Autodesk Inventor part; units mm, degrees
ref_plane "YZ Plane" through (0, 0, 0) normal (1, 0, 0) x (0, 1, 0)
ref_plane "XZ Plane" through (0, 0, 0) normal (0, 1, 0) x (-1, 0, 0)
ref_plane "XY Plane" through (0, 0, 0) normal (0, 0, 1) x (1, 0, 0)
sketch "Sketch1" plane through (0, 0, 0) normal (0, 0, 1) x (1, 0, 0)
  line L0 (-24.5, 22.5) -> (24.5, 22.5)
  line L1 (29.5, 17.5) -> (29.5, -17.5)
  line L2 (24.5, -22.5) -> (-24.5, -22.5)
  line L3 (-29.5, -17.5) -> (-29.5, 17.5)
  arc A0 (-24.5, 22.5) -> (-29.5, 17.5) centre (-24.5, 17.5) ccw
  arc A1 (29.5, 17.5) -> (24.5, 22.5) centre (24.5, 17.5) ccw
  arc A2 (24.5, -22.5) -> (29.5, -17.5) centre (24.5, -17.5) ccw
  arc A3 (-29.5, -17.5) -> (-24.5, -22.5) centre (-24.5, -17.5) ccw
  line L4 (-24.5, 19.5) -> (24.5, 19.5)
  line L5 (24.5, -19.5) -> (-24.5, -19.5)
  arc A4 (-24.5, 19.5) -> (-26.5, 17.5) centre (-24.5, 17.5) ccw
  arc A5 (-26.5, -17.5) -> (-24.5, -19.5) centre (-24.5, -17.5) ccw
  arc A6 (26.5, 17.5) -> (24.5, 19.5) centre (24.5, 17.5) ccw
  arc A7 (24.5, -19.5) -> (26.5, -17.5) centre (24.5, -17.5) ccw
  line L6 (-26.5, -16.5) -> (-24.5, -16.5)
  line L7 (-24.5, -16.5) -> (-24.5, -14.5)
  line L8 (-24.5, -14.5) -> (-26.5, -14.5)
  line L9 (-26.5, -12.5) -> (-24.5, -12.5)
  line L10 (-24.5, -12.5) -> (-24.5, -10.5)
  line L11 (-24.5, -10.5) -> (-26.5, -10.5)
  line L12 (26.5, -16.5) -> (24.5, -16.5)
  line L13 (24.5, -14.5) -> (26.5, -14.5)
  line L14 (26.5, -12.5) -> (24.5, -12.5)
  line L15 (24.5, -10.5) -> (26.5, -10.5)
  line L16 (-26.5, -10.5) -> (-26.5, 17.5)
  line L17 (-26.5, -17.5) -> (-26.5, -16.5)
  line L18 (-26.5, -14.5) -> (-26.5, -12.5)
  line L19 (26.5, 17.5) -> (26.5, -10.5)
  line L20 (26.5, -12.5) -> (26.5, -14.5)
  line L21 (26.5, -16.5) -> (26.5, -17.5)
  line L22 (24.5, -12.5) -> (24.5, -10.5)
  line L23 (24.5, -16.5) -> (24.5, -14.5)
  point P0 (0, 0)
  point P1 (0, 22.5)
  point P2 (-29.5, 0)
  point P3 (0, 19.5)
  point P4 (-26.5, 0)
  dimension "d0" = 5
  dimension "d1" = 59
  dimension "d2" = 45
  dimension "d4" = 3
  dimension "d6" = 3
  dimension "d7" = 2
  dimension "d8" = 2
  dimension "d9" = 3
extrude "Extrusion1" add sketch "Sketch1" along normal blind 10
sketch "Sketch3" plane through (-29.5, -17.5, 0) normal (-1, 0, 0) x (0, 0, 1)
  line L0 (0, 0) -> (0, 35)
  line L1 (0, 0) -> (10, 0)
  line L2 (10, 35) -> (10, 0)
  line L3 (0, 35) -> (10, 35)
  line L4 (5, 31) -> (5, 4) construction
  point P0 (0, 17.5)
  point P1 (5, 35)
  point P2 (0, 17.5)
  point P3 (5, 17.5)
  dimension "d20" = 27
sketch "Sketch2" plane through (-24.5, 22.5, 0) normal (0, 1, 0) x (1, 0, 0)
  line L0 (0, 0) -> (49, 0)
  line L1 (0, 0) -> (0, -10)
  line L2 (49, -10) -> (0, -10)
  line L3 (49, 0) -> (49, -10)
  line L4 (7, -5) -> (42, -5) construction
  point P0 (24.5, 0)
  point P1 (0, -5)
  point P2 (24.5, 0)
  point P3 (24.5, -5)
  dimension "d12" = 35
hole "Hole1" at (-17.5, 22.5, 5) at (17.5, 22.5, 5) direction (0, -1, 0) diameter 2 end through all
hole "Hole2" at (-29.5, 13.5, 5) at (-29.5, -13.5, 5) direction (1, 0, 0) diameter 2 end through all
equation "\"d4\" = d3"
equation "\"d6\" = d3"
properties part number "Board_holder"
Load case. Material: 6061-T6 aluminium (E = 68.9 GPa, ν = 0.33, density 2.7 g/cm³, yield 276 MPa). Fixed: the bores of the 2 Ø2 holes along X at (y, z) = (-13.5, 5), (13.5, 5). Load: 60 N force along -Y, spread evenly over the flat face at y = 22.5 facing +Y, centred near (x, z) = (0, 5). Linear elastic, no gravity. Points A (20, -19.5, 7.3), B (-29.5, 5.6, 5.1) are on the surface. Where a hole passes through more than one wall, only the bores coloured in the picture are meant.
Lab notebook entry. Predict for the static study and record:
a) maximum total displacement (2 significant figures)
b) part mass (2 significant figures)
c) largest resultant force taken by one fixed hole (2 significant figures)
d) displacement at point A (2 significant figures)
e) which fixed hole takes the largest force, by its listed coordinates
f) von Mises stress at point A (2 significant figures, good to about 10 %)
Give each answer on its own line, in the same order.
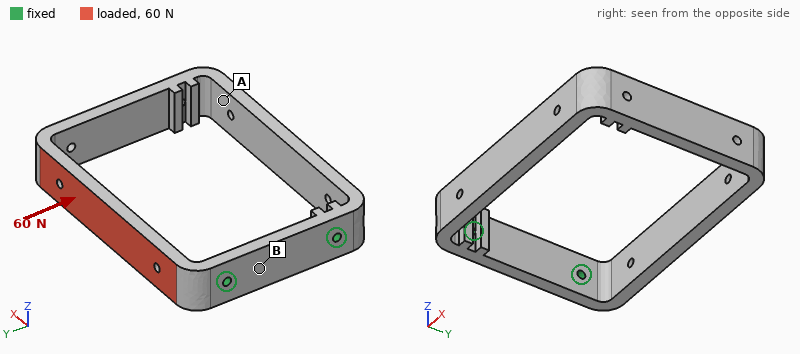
0.26 mm
16 g
49 N
0.23 mm
(13.5, 5)
19 MPa
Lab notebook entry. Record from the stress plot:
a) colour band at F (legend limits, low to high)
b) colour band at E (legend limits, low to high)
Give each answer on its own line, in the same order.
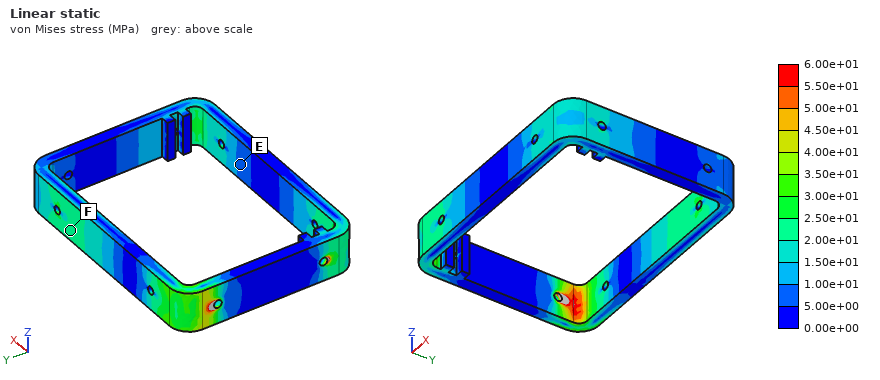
2.00e+01 to 2.50e+01 MPa
5.00e+00 to 1.00e+01 MPa
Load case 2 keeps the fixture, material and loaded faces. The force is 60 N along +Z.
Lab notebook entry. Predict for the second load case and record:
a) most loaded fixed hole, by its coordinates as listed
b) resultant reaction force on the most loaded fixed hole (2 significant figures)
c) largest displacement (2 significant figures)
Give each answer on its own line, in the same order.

(13.5, 5)
73 N
0.25 mm
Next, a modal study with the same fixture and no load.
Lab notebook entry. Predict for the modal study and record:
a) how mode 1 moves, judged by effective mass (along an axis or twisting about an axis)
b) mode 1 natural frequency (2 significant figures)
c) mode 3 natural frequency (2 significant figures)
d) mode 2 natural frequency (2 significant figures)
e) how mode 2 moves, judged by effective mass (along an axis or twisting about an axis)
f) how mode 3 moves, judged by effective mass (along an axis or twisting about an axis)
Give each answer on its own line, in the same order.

along Y
680 Hz
1600 Hz
810 Hz
along Z
twisting about X
